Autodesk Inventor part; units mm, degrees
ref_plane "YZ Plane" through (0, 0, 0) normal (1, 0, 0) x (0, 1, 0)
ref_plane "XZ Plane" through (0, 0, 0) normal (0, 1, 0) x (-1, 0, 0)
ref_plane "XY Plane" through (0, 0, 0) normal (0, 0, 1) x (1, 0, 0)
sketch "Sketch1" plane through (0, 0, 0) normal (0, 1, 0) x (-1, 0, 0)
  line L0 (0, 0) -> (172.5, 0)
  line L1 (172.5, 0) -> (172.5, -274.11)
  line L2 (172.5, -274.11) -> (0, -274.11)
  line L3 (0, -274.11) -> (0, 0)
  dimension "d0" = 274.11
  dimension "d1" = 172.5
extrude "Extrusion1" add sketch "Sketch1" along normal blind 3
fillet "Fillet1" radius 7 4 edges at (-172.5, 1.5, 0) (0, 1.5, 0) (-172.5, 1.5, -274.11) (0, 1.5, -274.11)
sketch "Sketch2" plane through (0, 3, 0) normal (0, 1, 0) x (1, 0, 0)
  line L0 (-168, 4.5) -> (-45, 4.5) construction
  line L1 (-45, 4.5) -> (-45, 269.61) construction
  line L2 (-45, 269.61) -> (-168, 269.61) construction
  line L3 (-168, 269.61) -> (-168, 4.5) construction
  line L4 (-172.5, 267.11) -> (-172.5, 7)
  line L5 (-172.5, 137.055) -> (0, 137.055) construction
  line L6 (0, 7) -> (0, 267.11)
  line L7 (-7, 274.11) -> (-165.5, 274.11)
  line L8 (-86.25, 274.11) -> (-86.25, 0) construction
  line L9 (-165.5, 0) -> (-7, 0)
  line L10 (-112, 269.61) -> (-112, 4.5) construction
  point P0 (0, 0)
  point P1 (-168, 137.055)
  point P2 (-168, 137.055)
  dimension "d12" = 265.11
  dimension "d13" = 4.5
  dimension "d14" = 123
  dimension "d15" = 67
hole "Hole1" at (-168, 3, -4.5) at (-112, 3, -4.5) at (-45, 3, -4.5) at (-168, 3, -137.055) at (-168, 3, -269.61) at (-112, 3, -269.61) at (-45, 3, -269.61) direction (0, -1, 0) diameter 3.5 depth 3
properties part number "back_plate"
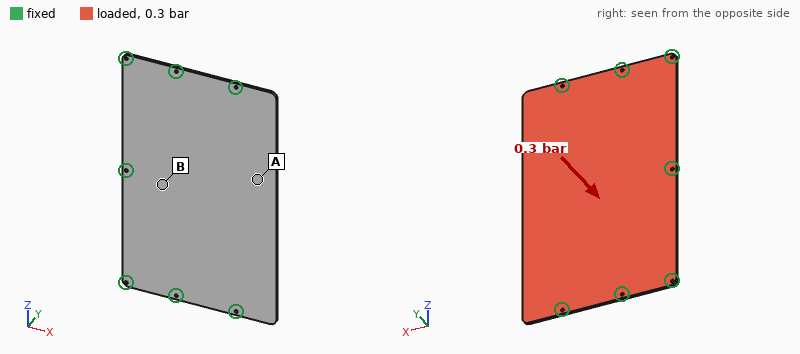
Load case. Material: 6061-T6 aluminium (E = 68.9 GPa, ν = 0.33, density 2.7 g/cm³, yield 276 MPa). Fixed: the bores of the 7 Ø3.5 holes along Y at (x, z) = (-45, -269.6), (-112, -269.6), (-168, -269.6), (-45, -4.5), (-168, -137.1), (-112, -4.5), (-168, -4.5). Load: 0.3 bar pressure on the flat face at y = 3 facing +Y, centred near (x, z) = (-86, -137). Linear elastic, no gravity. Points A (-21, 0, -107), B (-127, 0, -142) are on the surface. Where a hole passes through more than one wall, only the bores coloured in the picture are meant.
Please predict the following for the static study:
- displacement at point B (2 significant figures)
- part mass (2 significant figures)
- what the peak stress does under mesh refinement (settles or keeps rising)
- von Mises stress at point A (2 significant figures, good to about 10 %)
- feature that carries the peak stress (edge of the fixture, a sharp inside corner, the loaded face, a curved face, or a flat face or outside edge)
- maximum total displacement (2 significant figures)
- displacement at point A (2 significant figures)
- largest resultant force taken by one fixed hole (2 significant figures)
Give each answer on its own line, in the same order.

0.74 mm
380 g
keeps rising
48 MPa
edge of the fixture
3.5 mm
2.8 mm
380 N
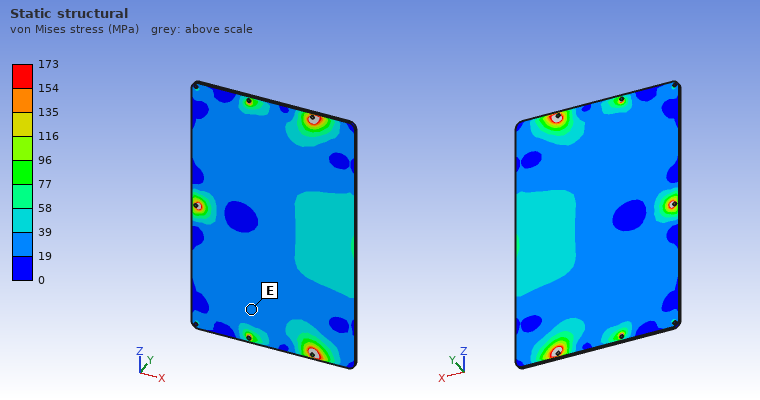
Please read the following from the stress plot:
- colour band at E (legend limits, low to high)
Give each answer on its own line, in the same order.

19 to 39 MPa
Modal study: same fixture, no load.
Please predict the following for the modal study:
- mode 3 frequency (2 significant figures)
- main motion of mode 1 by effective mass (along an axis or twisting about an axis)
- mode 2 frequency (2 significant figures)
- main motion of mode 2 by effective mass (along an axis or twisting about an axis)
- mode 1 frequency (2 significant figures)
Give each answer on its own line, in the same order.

570 Hz
along Y
540 Hz
twisting about X
220 Hz
